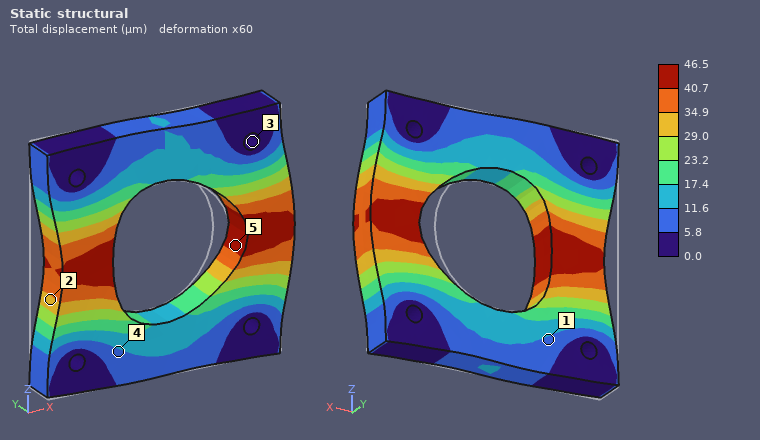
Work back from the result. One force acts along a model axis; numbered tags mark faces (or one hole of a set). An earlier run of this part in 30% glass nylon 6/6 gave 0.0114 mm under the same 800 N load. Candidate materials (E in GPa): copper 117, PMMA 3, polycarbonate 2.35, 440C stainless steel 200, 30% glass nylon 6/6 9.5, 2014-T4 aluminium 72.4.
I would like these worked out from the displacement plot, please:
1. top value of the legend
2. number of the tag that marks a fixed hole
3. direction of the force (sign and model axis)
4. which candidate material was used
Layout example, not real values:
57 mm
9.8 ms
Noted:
46.5 µm
3
+X
polycarbonate
